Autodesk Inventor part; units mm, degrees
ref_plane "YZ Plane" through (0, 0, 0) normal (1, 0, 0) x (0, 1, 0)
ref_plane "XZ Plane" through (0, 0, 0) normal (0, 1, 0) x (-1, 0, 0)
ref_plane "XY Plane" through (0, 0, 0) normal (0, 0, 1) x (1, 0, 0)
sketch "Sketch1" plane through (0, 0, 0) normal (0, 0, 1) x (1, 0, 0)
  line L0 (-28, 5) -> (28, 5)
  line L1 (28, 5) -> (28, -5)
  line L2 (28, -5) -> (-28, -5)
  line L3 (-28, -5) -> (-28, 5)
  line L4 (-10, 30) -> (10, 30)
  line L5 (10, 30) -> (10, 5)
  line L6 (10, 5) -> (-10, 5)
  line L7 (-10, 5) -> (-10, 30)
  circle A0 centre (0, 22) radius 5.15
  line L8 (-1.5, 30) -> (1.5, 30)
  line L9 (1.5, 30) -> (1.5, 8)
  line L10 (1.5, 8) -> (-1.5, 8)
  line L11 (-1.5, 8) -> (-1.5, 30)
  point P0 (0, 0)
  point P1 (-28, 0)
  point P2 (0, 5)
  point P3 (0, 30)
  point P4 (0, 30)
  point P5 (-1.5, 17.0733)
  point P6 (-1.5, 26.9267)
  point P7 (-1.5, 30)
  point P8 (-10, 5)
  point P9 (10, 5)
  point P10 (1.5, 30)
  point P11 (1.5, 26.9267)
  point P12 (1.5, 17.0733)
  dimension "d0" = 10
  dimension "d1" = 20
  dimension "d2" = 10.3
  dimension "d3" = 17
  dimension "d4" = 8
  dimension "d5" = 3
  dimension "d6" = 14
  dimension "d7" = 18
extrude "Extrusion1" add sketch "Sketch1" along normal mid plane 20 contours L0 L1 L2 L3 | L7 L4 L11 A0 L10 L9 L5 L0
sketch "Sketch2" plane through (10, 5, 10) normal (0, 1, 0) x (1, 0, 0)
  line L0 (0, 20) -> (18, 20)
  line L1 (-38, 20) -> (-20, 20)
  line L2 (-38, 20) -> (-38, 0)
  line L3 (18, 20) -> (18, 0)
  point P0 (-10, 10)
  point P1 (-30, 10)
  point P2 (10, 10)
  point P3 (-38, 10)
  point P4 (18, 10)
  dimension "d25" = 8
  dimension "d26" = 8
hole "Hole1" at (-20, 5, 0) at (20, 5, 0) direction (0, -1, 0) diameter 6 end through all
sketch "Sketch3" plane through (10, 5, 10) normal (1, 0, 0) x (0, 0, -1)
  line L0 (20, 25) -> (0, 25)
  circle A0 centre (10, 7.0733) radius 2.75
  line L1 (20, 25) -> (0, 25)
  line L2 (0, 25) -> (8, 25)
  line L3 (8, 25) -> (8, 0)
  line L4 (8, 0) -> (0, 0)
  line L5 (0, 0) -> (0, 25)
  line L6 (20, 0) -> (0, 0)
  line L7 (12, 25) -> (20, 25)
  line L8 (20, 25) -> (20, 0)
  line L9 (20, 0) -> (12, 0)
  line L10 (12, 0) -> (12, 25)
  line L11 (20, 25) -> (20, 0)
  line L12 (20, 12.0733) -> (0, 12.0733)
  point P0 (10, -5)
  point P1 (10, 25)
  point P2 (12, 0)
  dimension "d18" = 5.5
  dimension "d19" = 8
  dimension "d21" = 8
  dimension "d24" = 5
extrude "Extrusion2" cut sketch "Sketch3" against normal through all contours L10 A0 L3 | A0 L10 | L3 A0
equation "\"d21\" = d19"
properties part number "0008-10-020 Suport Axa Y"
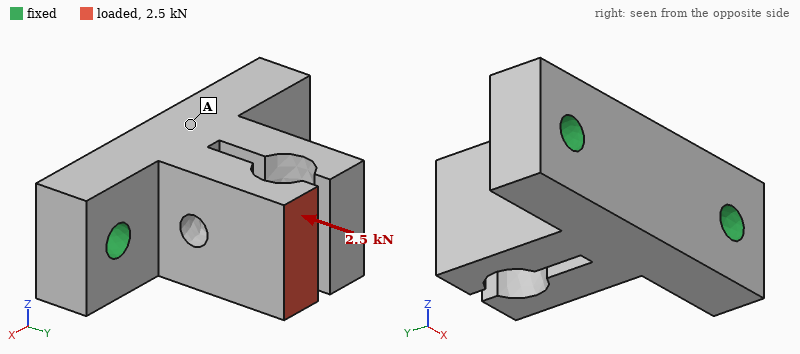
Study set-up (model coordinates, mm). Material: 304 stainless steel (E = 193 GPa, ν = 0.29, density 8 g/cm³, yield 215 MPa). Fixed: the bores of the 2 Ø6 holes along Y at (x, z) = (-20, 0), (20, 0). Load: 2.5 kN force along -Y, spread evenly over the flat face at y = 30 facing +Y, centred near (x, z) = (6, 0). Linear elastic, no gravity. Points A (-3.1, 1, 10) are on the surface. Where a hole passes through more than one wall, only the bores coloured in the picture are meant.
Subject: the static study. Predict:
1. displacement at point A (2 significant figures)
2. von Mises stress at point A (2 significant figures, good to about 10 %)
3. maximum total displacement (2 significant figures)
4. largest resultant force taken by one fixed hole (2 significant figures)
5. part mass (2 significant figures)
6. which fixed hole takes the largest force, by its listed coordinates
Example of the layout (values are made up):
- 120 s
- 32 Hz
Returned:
- 2.2 µm
- 9.6 MPa
- 13 µm
- 1.8 kN
- 140 g
- (20, 0)
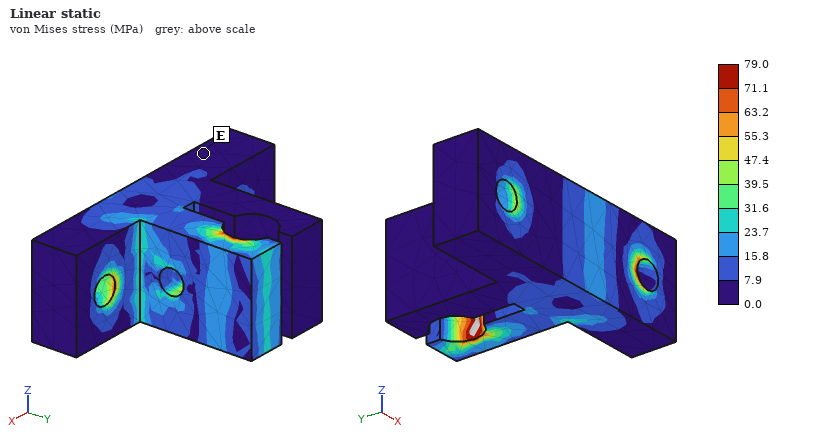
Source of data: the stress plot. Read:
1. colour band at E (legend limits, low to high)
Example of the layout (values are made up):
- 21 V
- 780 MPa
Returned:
- 0.0 to 7.9 MPa
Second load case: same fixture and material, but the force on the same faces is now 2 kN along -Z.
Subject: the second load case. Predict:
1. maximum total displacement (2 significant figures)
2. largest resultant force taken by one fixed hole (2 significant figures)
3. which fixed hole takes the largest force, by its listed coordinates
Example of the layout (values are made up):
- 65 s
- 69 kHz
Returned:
- 59 µm
- 1.3 kN
- (20, 0)
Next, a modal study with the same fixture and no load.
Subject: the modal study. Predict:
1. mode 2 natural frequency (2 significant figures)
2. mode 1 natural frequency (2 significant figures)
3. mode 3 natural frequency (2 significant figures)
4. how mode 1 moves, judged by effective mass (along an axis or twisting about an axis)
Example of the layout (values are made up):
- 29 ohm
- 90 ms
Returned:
- 8500 Hz
- 7300 Hz
- 8600 Hz
- along Z
